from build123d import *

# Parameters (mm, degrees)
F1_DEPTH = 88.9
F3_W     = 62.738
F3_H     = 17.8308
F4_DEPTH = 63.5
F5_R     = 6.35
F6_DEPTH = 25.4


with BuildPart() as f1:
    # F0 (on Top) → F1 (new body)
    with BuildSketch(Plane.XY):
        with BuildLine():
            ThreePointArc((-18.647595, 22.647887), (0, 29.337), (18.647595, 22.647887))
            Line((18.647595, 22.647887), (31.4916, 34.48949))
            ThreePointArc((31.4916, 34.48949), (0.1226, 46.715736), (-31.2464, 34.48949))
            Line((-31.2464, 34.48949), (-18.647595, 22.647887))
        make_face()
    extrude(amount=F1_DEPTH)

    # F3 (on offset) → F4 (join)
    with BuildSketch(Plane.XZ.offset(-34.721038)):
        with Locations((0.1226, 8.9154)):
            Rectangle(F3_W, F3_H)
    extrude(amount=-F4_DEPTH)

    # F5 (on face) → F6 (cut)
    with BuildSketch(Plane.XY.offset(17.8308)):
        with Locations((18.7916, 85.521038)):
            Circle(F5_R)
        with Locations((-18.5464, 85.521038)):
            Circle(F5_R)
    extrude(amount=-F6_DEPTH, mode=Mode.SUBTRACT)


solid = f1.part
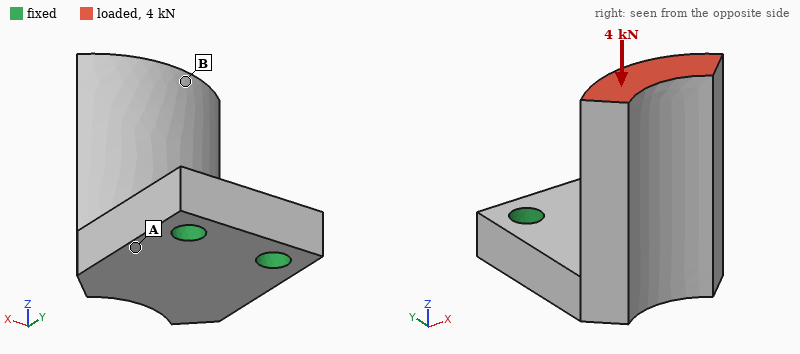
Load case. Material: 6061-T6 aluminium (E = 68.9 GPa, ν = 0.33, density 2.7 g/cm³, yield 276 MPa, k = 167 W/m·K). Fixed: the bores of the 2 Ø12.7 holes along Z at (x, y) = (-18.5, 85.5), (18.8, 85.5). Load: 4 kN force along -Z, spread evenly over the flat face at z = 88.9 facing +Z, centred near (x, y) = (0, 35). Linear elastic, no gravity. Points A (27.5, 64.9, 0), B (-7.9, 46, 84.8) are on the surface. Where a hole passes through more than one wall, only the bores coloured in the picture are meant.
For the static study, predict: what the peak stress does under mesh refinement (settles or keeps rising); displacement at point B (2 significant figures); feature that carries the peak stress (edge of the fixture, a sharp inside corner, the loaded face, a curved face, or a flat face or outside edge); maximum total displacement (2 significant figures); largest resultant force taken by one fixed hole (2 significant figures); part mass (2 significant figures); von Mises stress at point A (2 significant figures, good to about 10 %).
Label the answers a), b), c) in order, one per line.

a) keeps rising
b) 0.17 mm
c) edge of the fixture
d) 0.21 mm
e) 2.0 kN
f) 380 g
g) 36 MPa
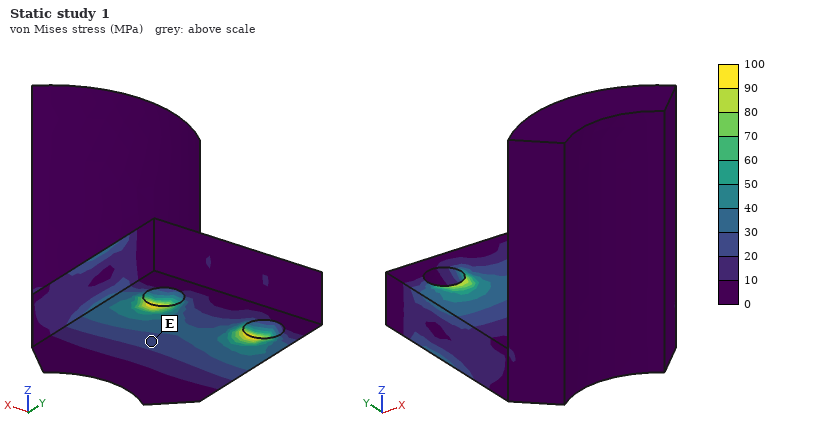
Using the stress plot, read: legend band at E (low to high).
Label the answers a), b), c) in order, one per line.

a) 20 to 30 MPa
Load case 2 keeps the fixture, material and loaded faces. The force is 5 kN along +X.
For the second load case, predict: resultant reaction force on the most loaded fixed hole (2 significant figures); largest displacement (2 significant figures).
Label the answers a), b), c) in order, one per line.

a) 10 kN
b) 0.48 mm
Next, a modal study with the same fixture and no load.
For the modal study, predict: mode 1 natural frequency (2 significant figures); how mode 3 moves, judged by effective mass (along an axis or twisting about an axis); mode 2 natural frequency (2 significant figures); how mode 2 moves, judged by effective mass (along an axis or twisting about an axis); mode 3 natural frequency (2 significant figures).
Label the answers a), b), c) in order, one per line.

a) 1300 Hz
b) along Z
c) 1900 Hz
d) along X
e) 3600 Hz
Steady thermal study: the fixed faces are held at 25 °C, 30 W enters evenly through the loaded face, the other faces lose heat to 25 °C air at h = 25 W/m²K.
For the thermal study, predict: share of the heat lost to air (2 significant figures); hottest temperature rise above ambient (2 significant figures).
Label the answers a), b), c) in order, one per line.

a) 14 %
b) 19 K
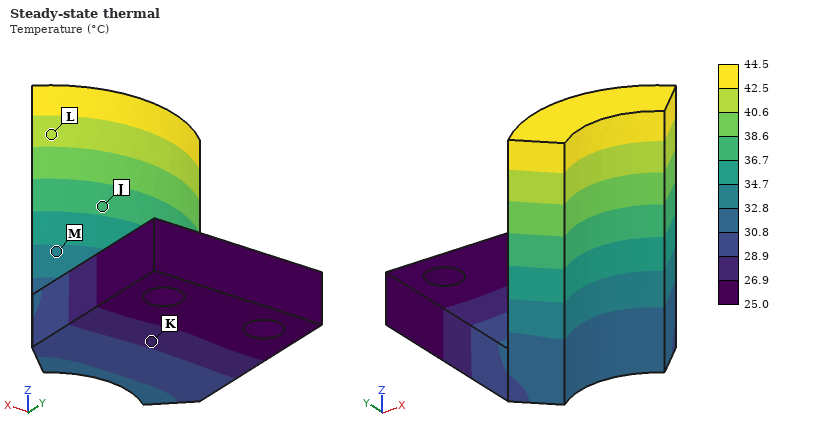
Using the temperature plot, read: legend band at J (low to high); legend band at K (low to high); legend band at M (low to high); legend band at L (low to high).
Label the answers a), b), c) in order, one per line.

a) 36.7 to 38.6 °C
b) 26.9 to 28.9 °C
c) 32.8 to 34.7 °C
d) 40.6 to 42.5 °C
